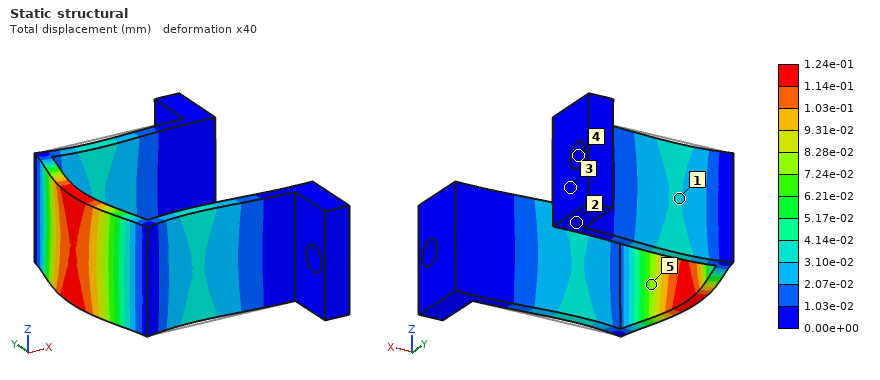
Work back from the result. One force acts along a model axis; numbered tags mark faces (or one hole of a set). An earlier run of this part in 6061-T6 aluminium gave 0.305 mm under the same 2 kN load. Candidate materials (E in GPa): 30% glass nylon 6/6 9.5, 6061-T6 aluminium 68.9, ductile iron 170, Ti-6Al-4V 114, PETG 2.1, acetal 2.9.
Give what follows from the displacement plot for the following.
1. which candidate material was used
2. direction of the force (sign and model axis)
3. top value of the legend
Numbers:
ductile iron
-X
1.24e-01 mm
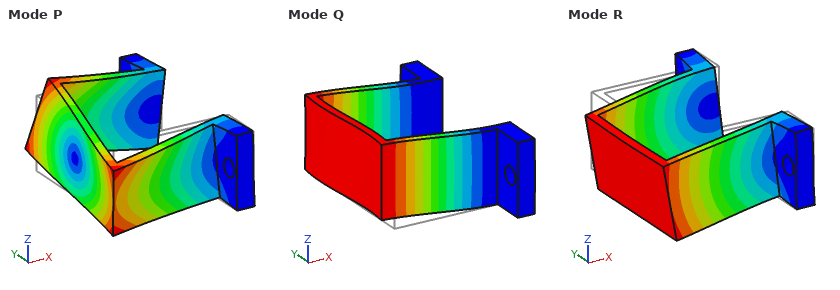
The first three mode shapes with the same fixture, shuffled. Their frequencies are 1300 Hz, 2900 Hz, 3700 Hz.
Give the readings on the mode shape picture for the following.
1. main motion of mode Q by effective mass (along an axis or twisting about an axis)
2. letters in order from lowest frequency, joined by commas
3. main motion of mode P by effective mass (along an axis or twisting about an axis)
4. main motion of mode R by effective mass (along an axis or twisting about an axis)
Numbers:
along Y
Q, R, P
twisting about X
along Z
